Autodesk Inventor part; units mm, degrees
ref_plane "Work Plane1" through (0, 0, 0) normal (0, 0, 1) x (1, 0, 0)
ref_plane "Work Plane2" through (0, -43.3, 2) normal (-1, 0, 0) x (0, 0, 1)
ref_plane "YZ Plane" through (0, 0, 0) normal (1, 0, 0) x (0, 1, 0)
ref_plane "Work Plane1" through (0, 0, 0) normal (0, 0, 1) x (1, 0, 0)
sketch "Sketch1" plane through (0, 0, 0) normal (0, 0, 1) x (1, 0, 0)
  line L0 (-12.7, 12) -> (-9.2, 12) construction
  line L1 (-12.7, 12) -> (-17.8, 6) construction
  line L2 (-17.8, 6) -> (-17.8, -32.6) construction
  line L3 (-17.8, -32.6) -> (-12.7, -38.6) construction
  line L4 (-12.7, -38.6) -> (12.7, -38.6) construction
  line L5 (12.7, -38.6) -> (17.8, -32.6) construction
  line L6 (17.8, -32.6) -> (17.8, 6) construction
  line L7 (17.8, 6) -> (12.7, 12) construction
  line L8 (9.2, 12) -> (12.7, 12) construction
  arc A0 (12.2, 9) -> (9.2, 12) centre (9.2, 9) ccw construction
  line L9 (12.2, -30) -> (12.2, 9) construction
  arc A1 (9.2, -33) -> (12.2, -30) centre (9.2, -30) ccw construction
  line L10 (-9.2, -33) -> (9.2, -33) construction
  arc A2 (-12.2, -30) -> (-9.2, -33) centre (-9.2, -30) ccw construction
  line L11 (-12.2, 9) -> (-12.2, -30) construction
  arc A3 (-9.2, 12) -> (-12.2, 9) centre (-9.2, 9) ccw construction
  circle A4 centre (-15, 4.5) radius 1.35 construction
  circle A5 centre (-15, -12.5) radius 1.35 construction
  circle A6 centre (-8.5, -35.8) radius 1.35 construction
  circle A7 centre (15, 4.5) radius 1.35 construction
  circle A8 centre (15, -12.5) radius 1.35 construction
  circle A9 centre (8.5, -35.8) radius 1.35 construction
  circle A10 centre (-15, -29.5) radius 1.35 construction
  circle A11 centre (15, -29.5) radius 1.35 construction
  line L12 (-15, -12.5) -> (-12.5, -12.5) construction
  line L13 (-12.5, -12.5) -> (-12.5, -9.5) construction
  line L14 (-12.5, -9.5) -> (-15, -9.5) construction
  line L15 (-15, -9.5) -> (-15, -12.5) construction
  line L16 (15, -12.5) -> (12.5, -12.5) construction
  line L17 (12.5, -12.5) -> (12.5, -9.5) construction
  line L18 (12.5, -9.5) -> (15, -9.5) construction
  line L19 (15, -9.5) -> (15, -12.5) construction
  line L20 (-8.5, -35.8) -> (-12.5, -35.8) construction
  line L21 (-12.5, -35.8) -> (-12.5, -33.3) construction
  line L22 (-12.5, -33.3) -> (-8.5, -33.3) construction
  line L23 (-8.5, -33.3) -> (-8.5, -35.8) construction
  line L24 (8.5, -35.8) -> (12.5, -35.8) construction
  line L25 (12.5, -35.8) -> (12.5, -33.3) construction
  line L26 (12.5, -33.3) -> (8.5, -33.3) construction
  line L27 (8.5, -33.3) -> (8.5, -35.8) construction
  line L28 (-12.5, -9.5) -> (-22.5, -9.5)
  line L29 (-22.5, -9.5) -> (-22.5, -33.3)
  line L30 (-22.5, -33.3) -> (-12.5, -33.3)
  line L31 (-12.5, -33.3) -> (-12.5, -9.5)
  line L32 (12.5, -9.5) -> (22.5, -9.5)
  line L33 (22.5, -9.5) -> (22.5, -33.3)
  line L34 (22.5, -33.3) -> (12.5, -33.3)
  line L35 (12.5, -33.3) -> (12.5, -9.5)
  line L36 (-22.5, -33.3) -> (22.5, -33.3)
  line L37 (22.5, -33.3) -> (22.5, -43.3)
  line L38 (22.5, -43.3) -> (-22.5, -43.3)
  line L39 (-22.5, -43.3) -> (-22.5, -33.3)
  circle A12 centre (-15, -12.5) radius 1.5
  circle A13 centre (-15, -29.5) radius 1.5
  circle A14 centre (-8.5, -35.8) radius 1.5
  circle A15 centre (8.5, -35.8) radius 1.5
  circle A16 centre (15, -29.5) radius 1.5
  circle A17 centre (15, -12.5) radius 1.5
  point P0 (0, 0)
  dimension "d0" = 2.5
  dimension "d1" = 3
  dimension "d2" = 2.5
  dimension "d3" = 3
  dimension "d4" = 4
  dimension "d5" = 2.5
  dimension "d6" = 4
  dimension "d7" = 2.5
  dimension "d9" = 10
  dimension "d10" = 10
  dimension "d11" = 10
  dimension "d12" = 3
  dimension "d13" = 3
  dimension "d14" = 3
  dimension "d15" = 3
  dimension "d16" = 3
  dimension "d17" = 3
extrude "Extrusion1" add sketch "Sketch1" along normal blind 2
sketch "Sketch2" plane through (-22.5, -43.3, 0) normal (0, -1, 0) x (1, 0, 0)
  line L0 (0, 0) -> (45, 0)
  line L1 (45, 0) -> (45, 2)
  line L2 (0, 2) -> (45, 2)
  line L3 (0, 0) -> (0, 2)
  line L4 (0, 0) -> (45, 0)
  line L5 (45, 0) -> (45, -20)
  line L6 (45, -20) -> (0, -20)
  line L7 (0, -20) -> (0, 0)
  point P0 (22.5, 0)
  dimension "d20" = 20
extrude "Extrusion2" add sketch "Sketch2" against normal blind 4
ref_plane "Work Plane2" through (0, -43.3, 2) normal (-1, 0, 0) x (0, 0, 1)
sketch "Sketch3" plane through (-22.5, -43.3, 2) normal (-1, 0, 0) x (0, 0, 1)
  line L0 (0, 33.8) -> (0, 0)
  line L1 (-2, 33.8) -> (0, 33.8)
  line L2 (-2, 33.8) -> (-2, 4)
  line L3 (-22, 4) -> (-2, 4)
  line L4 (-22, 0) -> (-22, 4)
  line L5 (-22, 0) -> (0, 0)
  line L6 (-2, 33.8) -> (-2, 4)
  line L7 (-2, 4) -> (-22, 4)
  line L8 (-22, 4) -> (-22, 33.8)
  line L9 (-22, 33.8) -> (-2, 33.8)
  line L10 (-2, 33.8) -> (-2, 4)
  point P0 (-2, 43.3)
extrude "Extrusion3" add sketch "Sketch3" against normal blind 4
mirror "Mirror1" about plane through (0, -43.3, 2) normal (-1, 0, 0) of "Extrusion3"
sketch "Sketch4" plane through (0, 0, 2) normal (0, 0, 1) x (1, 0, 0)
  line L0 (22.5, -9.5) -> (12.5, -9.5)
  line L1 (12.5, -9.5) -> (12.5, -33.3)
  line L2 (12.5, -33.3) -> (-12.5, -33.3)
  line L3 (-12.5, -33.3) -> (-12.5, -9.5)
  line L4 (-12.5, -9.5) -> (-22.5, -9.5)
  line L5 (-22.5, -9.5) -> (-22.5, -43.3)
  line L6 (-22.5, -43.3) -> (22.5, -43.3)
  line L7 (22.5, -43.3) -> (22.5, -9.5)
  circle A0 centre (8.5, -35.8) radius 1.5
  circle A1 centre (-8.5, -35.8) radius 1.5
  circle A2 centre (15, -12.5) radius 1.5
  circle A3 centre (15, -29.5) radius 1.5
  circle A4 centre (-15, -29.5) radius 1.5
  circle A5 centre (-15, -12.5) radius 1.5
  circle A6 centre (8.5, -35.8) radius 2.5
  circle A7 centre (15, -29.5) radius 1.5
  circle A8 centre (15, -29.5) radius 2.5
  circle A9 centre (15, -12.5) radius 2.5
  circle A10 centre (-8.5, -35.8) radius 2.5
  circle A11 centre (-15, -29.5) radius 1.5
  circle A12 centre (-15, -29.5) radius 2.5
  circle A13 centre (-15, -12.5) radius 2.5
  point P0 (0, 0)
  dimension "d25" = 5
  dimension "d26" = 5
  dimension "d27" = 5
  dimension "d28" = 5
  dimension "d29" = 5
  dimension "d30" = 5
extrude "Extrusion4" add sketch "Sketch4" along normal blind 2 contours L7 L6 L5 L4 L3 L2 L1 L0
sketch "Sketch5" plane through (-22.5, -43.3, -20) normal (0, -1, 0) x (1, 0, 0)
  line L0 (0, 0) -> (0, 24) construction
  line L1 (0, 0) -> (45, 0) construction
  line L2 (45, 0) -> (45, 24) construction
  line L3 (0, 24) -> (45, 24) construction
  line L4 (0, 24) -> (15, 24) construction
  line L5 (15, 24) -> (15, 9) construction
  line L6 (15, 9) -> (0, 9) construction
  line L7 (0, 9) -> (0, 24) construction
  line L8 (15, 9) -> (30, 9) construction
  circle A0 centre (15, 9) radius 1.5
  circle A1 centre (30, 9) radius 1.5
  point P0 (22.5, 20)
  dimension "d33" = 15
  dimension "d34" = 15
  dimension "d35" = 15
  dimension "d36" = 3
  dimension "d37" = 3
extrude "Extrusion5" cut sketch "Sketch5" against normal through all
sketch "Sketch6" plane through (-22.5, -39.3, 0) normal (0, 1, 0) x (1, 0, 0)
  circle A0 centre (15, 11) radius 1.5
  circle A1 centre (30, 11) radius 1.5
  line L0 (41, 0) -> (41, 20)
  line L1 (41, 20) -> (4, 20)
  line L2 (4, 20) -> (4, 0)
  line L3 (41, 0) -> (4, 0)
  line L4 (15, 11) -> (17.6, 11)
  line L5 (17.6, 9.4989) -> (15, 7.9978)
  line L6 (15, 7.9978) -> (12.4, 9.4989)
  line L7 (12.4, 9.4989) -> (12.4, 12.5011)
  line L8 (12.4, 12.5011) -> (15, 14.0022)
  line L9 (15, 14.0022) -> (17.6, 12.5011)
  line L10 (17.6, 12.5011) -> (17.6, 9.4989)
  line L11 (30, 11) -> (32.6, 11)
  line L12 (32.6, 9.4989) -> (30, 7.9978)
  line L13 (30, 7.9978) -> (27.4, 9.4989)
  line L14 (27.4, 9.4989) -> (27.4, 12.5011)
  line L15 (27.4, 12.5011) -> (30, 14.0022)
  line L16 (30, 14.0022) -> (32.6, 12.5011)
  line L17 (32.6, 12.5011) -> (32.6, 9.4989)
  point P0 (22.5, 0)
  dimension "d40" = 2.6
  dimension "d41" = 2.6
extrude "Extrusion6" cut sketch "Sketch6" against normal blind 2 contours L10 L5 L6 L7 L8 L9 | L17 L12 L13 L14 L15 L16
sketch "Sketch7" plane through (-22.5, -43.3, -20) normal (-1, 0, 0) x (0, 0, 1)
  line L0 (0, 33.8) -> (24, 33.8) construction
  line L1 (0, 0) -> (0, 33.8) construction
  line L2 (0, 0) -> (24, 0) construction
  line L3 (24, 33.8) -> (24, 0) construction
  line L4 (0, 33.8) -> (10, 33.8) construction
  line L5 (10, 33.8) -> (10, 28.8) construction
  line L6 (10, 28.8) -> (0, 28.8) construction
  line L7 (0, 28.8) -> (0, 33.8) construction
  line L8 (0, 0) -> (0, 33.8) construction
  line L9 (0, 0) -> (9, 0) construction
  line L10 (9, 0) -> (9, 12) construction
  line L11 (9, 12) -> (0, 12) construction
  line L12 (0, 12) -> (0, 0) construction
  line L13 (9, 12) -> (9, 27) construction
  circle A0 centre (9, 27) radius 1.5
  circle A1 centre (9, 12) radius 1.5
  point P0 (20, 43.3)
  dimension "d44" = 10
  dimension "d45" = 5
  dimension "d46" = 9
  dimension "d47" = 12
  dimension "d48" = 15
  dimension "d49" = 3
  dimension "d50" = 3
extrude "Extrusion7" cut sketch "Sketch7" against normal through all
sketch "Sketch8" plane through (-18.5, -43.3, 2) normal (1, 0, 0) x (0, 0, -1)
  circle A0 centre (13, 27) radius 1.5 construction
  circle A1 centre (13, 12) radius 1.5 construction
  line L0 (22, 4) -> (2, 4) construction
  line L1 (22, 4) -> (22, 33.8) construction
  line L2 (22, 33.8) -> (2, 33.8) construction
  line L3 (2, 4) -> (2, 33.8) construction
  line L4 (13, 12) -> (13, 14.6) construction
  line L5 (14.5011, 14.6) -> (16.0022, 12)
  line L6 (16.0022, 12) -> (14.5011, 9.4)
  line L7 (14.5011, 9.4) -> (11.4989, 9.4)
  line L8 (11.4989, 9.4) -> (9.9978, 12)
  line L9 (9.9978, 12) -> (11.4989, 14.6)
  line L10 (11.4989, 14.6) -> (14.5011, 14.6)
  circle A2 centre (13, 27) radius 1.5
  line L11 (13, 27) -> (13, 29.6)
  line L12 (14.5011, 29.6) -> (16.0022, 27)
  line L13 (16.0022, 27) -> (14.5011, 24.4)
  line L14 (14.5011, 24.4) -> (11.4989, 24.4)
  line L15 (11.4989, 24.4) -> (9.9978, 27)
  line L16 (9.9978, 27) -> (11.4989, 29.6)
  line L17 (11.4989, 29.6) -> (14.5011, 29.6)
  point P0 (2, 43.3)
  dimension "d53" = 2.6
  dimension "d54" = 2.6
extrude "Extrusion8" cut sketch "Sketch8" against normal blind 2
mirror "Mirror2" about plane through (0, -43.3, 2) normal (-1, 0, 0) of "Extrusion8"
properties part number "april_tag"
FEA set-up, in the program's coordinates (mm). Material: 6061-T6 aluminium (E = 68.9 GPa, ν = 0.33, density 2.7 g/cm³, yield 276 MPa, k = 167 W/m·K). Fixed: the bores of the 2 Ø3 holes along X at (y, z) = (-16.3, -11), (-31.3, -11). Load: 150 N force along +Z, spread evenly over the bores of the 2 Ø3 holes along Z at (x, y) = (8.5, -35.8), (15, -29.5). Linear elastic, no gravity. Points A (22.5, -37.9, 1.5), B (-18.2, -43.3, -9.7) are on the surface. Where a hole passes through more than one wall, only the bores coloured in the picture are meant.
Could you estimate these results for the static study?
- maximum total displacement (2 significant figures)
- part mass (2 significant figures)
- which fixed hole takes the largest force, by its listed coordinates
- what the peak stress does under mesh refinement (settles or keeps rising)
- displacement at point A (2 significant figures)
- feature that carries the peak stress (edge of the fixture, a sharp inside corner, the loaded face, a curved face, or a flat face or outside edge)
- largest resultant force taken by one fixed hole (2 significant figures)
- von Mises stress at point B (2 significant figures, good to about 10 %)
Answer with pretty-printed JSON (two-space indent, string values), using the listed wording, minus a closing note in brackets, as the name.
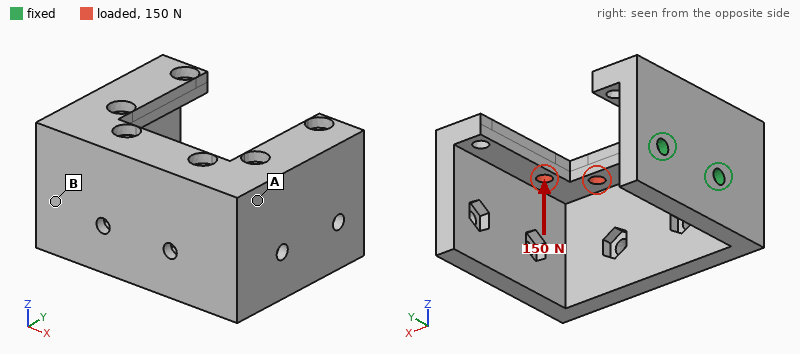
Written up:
{
  "maximum total displacement": "0.41 mm",
  "part mass": "31 g",
  "which fixed hole takes the largest force, by its listed coordinates": "(-31.3, -11)",
  "what the peak stress does under mesh refinement": "keeps rising",
  "displacement at point A": "0.32 mm",
  "feature that carries the peak stress": "edge of the fixture",
  "largest resultant force taken by one fixed hole": "140 N",
  "von Mises stress at point B": "28 MPa"
}
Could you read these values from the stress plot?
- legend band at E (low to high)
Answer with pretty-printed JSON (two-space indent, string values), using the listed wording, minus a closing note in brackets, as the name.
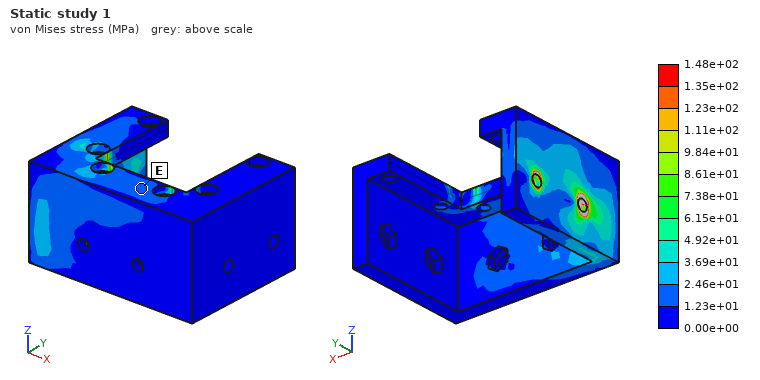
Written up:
{
  "legend band at E": "1.23e+01 to 2.46e+01 MPa"
}
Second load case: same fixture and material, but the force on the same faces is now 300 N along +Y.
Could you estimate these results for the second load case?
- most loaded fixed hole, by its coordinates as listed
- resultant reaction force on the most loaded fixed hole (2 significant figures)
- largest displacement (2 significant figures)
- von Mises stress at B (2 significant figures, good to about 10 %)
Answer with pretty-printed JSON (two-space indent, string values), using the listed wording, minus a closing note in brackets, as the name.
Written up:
{
  "most loaded fixed hole, by its coordinates as listed": "(-16.3, -11)",
  "resultant reaction force on the most loaded fixed hole": "740 N",
  "largest displacement": "0.55 mm",
  "von Mises stress at B": "33 MPa"
}
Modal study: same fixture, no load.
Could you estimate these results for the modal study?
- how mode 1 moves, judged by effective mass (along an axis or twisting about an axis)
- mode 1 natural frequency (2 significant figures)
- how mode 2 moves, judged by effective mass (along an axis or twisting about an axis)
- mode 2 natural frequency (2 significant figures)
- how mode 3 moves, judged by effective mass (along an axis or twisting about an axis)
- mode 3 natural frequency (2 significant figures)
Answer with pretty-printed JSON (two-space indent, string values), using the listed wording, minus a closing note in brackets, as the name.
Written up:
{
  "how mode 1 moves, judged by effective mass": "along Z",
  "mode 1 natural frequency": "800 Hz",
  "how mode 2 moves, judged by effective mass": "along Y",
  "mode 2 natural frequency": "980 Hz",
  "how mode 3 moves, judged by effective mass": "along X",
  "mode 3 natural frequency": "2400 Hz"
}
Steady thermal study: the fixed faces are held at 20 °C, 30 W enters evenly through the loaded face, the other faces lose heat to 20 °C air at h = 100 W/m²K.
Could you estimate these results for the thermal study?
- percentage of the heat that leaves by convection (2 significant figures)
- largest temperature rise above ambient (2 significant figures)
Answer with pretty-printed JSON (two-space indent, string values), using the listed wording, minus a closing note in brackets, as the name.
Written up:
{
  "percentage of the heat that leaves by convection": "57 %",
  "largest temperature rise above ambient": "58 K"
}
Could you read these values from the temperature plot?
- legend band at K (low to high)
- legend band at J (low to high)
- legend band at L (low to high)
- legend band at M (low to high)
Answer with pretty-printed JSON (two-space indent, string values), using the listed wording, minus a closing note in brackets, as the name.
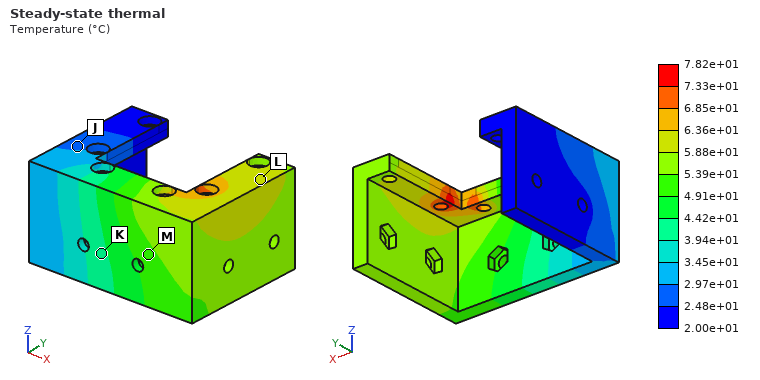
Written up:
{
  "legend band at K": "3.94e+01 to 4.42e+01 °C",
  "legend band at J": "2.48e+01 to 2.97e+01 °C",
  "legend band at L": "5.88e+01 to 6.36e+01 °C",
  "legend band at M": "4.91e+01 to 5.39e+01 °C"
}
